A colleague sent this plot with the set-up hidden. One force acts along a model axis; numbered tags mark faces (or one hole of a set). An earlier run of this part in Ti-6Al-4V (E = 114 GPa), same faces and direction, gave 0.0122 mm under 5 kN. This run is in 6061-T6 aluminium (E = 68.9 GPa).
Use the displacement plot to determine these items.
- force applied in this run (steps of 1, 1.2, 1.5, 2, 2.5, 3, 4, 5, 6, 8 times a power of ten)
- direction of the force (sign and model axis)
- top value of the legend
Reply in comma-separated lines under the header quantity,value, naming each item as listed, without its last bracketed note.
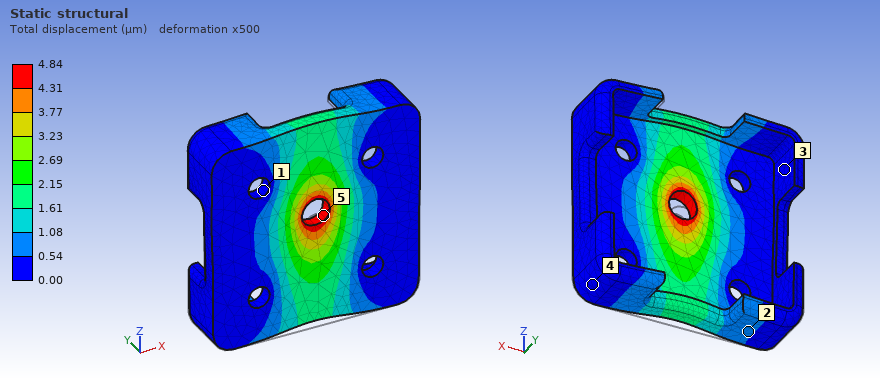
quantity,value
force applied in this run,1.2 kN
direction of the force,+Z
top value of the legend,4.84 µm
